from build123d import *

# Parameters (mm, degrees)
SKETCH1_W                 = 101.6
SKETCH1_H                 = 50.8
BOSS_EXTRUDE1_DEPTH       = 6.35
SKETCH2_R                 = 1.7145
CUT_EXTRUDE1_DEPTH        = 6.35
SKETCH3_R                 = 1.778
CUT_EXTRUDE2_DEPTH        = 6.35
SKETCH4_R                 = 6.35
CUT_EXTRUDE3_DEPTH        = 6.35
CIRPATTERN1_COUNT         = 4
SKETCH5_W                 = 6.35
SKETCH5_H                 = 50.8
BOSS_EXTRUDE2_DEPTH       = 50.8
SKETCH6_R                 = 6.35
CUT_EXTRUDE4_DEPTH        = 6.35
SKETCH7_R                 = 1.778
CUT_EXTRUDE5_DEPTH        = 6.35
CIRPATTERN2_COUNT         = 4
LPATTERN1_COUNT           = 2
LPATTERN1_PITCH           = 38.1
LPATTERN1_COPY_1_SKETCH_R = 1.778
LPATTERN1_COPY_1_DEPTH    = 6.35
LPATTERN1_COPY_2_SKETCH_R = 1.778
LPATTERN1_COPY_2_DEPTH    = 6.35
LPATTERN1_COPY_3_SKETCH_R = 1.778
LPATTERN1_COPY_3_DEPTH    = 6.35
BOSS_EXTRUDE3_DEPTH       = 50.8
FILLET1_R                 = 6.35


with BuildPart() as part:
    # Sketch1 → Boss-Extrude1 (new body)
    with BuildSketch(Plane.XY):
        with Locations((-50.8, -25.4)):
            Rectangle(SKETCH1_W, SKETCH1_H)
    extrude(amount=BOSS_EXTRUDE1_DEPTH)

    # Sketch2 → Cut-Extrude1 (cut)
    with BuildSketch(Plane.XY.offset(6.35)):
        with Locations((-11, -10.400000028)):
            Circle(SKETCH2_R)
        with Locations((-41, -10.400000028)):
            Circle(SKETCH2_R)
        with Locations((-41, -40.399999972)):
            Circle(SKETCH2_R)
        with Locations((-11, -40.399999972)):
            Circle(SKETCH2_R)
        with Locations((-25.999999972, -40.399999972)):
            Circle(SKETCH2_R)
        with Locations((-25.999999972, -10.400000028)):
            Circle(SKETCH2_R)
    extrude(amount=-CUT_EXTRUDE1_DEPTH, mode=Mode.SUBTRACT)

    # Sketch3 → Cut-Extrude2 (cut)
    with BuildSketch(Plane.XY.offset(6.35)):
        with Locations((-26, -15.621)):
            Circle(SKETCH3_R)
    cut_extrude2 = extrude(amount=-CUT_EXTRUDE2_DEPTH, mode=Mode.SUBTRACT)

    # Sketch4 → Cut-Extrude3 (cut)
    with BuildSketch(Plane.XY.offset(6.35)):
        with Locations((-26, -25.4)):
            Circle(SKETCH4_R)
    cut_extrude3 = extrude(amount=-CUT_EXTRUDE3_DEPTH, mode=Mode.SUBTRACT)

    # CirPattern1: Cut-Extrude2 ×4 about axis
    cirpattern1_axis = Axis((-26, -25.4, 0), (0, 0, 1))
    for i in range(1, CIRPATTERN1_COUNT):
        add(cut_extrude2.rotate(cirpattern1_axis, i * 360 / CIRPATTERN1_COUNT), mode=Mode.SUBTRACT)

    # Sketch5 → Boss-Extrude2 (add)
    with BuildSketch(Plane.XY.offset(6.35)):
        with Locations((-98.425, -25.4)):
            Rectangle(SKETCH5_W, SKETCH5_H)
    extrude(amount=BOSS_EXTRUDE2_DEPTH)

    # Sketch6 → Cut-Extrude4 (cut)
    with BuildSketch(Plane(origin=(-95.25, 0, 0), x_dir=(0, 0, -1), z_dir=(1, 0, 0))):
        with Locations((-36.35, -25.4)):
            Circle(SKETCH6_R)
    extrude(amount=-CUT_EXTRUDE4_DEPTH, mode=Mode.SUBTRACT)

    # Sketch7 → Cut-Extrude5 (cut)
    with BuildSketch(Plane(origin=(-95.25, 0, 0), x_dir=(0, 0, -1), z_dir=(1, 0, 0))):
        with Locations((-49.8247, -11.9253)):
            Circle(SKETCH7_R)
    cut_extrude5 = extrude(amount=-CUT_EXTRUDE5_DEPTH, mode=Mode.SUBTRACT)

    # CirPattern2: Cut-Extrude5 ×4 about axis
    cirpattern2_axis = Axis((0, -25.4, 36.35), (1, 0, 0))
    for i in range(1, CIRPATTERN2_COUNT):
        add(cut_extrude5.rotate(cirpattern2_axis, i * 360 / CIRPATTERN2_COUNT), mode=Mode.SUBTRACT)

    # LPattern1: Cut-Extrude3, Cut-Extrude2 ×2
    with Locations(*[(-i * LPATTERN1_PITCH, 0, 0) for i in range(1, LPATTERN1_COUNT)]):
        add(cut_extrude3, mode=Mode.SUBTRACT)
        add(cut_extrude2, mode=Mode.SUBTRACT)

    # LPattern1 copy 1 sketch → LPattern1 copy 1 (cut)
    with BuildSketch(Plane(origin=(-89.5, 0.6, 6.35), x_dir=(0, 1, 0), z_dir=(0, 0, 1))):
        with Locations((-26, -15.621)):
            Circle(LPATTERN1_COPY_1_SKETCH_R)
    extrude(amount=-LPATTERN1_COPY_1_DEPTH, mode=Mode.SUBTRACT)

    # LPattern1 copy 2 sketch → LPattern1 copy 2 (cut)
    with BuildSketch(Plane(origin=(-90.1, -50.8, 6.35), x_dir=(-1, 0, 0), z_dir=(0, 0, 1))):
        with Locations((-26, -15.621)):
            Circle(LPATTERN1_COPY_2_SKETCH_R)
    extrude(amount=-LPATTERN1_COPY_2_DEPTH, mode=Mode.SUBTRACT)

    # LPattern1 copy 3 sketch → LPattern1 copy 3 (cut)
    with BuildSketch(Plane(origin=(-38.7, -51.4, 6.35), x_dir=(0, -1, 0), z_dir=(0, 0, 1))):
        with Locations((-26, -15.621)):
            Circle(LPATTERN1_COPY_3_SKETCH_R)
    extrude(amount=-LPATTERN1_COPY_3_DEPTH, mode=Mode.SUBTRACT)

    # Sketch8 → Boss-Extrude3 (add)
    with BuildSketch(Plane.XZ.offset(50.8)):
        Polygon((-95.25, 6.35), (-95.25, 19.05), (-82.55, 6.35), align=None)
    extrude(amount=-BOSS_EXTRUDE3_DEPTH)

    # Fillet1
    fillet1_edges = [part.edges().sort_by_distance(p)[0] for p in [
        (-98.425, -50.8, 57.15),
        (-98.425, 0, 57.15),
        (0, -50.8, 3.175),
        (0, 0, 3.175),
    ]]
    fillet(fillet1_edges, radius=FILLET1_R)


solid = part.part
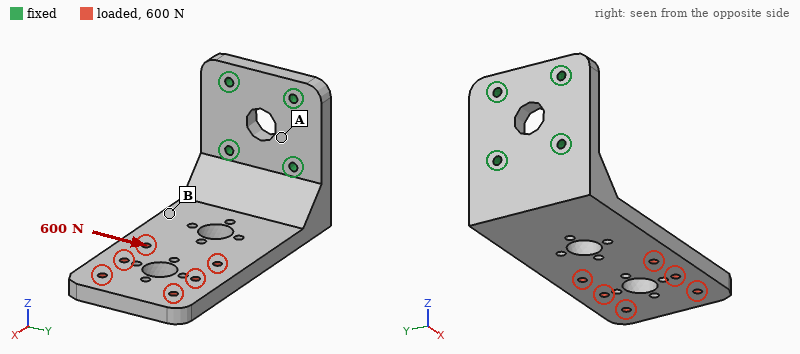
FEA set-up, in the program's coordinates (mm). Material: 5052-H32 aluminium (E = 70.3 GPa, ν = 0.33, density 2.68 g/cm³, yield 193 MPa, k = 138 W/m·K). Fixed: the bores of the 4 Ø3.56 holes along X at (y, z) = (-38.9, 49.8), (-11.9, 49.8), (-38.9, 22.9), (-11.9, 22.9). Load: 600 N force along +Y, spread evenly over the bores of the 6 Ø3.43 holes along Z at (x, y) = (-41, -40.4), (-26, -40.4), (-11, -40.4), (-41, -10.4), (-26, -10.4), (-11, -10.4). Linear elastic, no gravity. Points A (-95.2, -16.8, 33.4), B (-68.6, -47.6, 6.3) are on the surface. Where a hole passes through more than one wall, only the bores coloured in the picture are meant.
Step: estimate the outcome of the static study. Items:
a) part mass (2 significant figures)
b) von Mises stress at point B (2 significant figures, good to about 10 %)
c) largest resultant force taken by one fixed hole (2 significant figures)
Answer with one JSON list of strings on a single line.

["130 g", "15 MPa", "1.5 kN"]
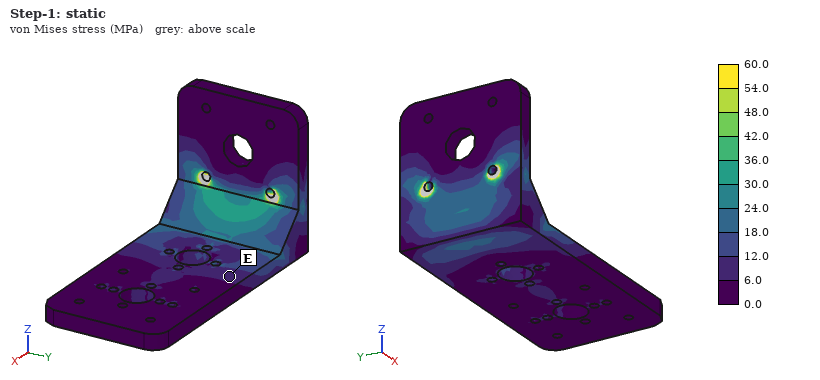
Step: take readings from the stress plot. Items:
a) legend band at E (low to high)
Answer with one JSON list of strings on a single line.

["6.0 to 12.0 MPa"]
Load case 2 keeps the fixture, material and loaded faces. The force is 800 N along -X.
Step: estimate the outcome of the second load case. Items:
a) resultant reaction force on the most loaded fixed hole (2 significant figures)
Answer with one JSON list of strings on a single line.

["500 N"]
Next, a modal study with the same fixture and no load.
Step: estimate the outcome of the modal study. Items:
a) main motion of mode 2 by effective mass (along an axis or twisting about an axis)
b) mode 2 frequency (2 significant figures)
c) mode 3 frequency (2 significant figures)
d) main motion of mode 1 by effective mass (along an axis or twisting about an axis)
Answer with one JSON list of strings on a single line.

["along Y", "1700 Hz", "2400 Hz", "along Z"]
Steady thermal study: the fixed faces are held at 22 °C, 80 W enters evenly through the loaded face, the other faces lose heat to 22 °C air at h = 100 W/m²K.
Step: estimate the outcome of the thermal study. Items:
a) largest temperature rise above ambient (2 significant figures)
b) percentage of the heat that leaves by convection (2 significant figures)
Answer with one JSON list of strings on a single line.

["73 K", "66 %"]
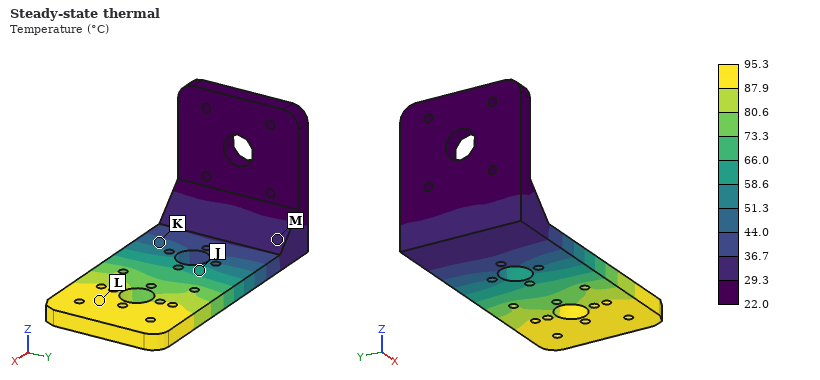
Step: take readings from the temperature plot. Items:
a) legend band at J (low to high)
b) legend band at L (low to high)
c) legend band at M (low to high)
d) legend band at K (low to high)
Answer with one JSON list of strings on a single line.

["58.6 to 66.0 °C", "87.9 to 95.3 °C", "29.3 to 36.7 °C", "44.0 to 51.3 °C"]
